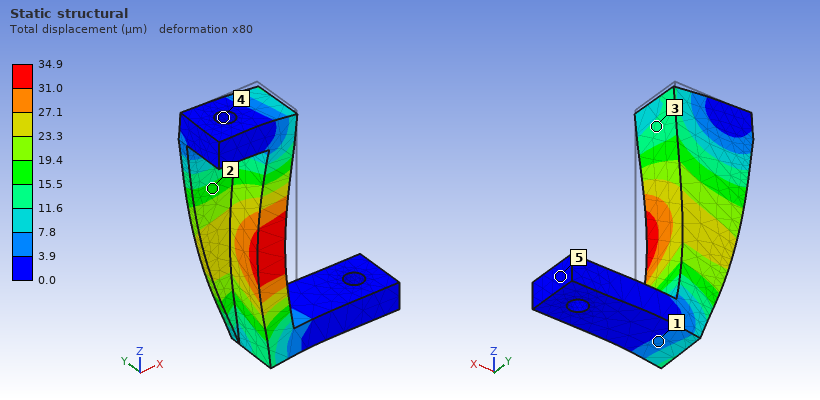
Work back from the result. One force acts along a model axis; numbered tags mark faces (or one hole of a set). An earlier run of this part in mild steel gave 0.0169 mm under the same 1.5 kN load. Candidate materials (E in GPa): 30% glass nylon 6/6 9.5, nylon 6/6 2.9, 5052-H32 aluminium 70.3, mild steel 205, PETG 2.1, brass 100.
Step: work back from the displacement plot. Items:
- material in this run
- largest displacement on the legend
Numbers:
brass
34.9 µm
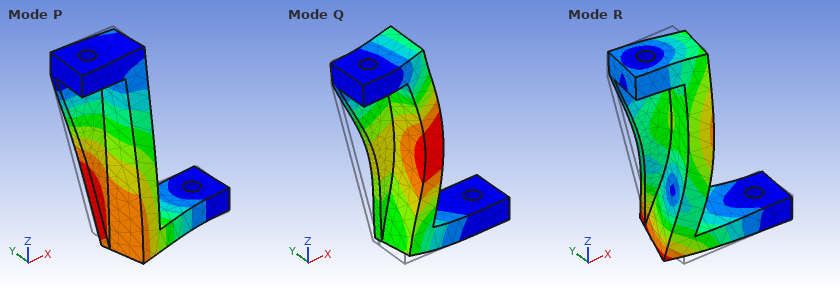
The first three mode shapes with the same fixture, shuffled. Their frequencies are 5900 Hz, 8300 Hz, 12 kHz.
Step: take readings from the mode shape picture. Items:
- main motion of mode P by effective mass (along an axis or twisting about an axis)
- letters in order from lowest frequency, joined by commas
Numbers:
along Y
P, Q, R
